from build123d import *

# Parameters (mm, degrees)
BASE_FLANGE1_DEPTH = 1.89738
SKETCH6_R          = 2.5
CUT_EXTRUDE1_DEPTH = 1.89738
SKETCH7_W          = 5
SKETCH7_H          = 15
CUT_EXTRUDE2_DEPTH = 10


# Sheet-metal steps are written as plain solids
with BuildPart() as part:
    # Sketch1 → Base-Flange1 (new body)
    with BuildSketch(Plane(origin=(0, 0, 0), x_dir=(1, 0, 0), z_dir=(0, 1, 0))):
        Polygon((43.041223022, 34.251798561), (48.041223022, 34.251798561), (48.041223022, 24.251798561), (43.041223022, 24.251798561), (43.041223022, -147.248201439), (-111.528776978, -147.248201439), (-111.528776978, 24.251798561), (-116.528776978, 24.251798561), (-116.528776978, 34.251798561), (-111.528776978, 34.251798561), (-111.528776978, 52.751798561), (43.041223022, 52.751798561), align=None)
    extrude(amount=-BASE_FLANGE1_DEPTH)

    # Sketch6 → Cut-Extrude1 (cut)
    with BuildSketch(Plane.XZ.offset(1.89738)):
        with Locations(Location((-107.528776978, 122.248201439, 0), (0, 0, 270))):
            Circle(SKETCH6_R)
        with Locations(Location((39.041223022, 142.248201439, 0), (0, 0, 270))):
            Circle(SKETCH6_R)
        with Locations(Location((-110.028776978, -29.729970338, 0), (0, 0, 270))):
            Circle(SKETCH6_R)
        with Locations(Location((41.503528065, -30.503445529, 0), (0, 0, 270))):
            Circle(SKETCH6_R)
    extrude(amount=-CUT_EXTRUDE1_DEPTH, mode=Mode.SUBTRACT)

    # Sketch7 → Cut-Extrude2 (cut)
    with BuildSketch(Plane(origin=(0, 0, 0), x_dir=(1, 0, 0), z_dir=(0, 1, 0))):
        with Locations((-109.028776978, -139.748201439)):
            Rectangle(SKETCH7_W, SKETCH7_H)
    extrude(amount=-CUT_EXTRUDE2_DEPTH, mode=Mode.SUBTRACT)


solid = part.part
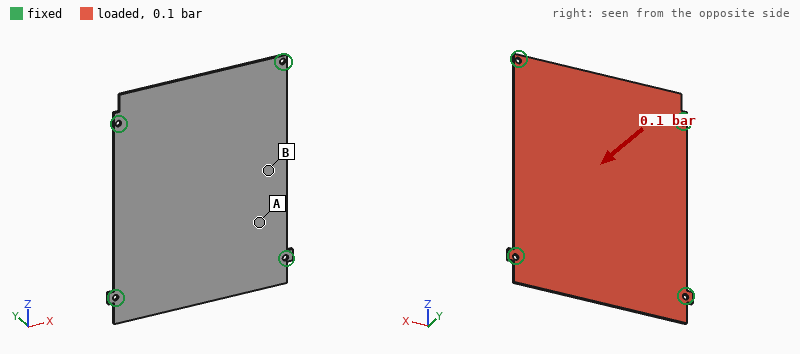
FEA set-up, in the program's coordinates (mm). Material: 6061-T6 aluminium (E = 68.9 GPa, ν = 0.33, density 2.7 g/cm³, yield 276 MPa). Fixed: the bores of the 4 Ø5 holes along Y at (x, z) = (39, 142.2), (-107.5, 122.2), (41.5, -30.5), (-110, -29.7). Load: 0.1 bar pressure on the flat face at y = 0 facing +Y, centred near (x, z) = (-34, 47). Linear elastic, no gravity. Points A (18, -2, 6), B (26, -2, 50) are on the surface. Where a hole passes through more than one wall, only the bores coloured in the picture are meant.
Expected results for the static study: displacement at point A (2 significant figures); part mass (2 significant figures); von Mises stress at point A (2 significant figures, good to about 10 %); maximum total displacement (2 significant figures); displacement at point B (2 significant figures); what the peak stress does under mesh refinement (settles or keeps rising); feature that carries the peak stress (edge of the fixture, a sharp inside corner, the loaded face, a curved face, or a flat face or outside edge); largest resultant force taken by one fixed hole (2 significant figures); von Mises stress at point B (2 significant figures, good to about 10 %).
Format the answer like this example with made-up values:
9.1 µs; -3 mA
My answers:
0.68 mm; 160 g; 15 MPa; 1.2 mm; 1.0 mm; keeps rising; edge of the fixture; 84 N; 28 MPa
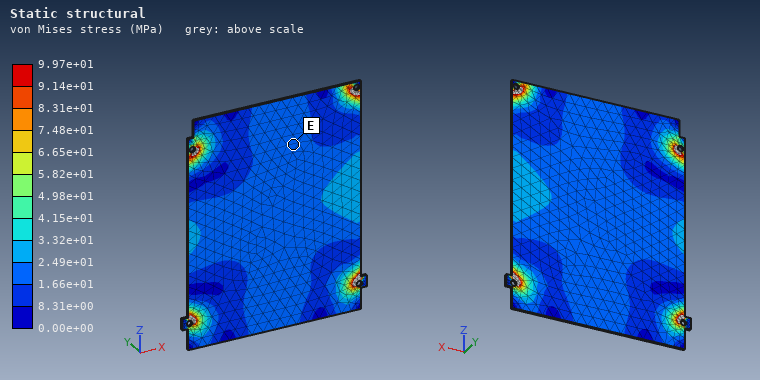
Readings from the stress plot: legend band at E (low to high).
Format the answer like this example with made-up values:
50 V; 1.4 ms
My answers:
1.66e+01 to 2.49e+01 MPa
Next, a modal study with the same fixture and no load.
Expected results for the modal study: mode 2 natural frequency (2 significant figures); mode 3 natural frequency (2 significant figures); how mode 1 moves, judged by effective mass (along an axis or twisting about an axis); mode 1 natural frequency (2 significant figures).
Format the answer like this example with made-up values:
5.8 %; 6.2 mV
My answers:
410 Hz; 450 Hz; along Y; 240 Hz
